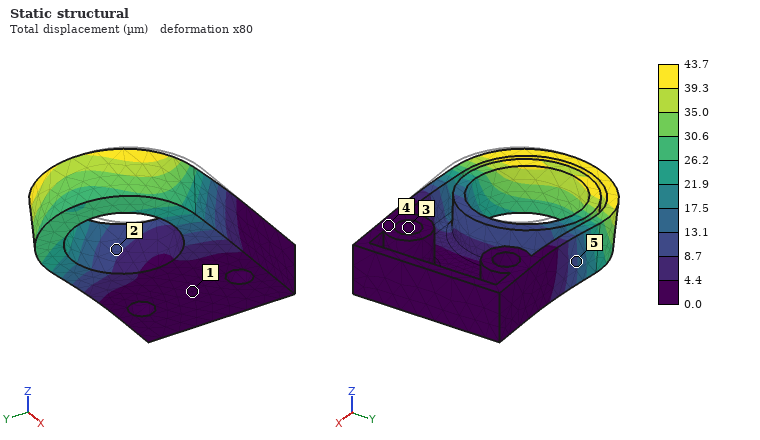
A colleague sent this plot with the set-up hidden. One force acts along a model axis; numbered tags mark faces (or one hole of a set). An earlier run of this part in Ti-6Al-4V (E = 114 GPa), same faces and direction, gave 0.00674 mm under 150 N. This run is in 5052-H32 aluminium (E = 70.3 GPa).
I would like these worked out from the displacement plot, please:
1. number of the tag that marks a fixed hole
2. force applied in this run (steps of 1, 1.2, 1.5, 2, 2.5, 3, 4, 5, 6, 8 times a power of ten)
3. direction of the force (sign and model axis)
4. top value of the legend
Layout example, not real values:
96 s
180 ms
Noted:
3
600 N
+Y
43.7 µm
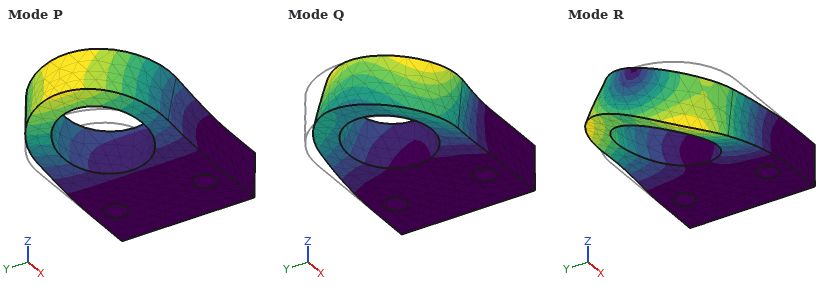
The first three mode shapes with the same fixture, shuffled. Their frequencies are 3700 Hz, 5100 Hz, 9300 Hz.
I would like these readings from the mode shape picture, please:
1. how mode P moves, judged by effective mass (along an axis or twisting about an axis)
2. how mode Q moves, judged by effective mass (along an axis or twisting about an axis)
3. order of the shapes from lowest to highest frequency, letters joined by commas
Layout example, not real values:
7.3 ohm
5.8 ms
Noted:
along Z
along Y
P, Q, R
